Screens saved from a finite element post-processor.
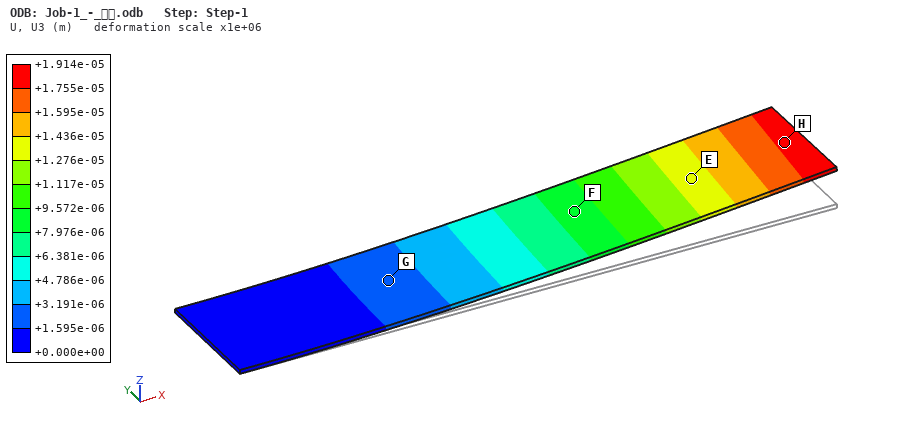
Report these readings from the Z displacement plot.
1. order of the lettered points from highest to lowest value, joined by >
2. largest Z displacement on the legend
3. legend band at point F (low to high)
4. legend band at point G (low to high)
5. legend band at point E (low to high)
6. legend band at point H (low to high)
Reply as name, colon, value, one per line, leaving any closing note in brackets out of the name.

order of the lettered points from highest to lowest value, joined by >: H > E > F > G
largest Z displacement on the legend: +1.914e-05 m
legend band at point F: +7.976e-06 to +9.572e-06 m
legend band at point G: +1.595e-06 to +3.191e-06 m
legend band at point E: +1.276e-05 to +1.436e-05 m
legend band at point H: +1.755e-05 to +1.914e-05 m
